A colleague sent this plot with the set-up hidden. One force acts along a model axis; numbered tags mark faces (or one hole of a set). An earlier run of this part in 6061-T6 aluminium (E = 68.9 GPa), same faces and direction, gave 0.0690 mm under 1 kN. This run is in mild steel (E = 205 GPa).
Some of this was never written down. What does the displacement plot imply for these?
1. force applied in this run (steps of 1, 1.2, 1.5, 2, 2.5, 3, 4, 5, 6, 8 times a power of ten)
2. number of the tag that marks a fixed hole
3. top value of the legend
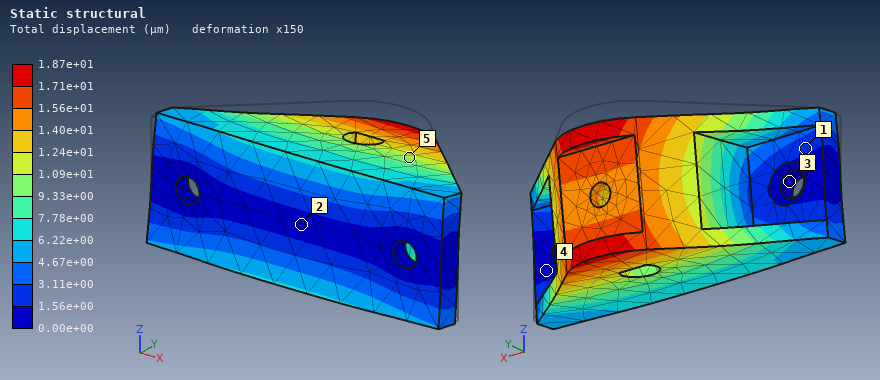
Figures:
800 N
3
1.87e+01 µm
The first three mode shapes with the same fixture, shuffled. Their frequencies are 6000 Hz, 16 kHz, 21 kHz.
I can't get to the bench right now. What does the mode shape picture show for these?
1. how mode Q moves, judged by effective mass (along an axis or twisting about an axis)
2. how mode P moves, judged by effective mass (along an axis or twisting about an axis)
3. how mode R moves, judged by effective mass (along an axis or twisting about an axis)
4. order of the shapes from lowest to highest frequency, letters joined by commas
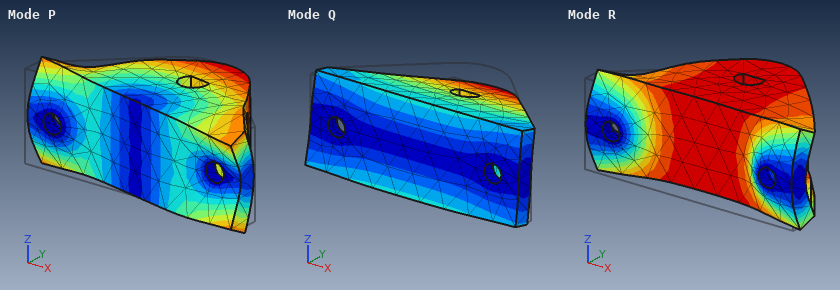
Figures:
along Z
along X
along Y
Q, R, P
